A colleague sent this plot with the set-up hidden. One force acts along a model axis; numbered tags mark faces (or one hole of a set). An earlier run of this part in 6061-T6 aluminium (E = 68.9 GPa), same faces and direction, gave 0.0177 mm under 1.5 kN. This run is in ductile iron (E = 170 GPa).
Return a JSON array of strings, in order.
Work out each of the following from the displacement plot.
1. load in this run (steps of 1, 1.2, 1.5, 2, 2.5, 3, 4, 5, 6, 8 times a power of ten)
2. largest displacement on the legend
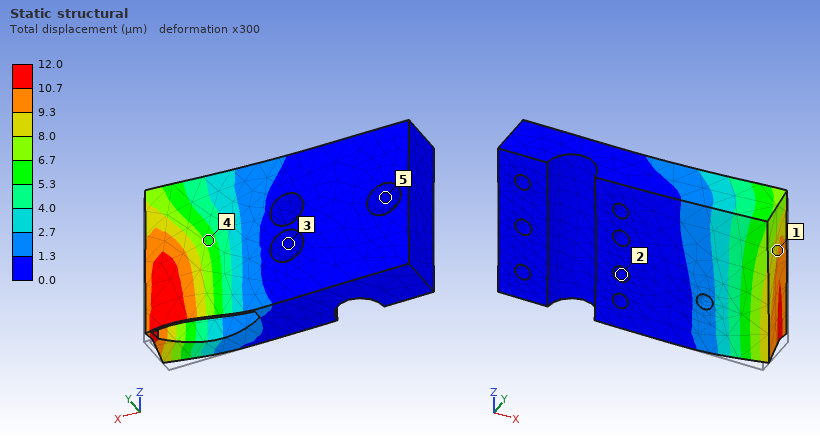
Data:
["2.5 kN", "12.0 µm"]
